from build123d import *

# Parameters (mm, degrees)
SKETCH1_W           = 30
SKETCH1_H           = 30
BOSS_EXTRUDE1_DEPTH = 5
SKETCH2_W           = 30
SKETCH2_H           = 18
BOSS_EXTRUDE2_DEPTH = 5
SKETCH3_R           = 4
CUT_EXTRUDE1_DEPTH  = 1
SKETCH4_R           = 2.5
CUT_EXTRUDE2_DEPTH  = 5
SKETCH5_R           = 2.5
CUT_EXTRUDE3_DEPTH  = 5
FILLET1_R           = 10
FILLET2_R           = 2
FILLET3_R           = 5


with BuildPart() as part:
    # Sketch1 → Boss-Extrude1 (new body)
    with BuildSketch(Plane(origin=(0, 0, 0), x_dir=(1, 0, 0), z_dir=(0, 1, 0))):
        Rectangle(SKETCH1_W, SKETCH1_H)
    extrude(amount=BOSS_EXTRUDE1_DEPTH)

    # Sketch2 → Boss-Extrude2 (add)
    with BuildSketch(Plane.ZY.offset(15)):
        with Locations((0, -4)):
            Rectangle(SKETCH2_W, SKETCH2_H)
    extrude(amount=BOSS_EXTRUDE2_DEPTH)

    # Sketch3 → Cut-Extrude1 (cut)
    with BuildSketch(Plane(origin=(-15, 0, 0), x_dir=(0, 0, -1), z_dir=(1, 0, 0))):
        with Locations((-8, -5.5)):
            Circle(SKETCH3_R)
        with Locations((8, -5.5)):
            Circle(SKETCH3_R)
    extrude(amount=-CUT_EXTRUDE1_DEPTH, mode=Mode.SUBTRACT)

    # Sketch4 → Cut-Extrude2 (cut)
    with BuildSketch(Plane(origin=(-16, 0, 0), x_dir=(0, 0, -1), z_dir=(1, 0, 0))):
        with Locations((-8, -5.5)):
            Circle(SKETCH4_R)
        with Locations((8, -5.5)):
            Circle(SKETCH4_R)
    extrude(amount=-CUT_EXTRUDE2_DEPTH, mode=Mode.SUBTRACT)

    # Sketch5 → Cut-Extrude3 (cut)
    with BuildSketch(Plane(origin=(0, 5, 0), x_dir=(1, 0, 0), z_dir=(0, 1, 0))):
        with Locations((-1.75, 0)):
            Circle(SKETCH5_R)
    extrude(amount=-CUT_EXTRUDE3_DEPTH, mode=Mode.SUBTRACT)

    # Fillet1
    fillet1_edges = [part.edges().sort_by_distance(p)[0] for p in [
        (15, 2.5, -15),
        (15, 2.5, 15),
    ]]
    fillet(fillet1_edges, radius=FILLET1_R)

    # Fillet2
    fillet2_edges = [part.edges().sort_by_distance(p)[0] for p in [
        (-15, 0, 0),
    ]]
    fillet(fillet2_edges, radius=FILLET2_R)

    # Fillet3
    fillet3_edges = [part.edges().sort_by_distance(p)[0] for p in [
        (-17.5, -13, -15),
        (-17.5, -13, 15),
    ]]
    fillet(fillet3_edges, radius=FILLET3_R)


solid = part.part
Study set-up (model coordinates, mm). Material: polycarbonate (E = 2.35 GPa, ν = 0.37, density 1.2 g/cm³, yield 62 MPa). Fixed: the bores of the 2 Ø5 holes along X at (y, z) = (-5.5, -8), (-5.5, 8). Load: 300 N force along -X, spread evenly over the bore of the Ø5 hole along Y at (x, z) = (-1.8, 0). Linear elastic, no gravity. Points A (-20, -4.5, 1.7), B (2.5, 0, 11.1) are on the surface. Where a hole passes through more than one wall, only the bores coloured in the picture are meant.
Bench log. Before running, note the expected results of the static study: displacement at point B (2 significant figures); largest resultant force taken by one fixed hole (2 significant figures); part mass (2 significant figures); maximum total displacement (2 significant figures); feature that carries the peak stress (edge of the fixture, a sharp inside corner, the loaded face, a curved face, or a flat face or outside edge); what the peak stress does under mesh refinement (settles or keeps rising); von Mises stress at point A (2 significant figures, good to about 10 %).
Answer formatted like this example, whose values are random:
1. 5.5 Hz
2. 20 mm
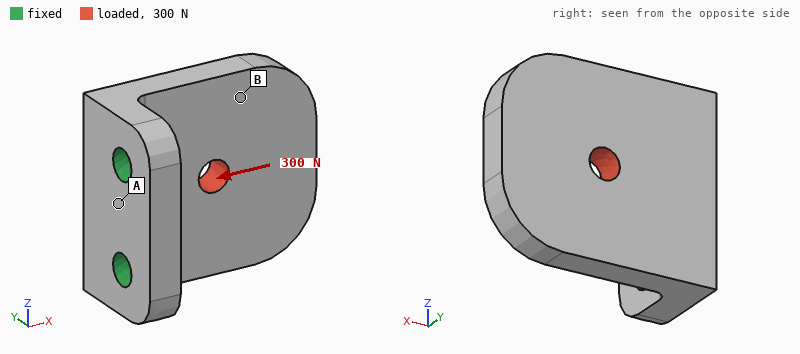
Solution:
1. 0.29 mm
2. 150 N
3. 7.9 g
4. 0.49 mm
5. edge of the fixture
6. keeps rising
7. 6.6 MPa
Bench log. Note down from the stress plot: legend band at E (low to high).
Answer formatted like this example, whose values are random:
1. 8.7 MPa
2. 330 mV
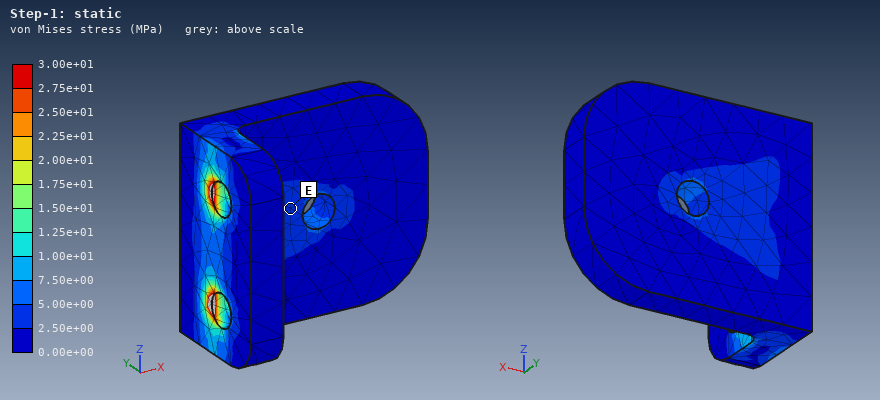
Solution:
1. 2.50e+00 to 5.00e+00 MPa
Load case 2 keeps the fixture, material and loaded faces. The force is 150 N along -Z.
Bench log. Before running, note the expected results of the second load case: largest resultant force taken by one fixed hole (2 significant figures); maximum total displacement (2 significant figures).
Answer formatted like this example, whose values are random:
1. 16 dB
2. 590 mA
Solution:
1. 160 N
2. 0.19 mm
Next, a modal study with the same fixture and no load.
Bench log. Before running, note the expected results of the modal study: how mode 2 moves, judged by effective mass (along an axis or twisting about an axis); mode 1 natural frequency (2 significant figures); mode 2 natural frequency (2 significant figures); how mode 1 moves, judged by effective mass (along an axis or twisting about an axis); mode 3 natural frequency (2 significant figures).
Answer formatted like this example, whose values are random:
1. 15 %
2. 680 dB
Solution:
1. along Z
2. 880 Hz
3. 2100 Hz
4. along Y
5. 3000 Hz
